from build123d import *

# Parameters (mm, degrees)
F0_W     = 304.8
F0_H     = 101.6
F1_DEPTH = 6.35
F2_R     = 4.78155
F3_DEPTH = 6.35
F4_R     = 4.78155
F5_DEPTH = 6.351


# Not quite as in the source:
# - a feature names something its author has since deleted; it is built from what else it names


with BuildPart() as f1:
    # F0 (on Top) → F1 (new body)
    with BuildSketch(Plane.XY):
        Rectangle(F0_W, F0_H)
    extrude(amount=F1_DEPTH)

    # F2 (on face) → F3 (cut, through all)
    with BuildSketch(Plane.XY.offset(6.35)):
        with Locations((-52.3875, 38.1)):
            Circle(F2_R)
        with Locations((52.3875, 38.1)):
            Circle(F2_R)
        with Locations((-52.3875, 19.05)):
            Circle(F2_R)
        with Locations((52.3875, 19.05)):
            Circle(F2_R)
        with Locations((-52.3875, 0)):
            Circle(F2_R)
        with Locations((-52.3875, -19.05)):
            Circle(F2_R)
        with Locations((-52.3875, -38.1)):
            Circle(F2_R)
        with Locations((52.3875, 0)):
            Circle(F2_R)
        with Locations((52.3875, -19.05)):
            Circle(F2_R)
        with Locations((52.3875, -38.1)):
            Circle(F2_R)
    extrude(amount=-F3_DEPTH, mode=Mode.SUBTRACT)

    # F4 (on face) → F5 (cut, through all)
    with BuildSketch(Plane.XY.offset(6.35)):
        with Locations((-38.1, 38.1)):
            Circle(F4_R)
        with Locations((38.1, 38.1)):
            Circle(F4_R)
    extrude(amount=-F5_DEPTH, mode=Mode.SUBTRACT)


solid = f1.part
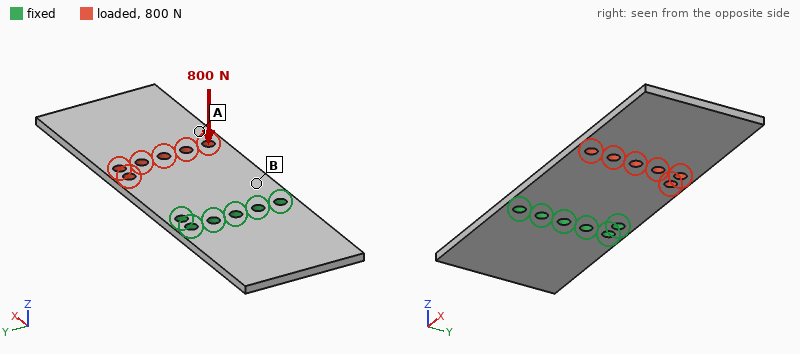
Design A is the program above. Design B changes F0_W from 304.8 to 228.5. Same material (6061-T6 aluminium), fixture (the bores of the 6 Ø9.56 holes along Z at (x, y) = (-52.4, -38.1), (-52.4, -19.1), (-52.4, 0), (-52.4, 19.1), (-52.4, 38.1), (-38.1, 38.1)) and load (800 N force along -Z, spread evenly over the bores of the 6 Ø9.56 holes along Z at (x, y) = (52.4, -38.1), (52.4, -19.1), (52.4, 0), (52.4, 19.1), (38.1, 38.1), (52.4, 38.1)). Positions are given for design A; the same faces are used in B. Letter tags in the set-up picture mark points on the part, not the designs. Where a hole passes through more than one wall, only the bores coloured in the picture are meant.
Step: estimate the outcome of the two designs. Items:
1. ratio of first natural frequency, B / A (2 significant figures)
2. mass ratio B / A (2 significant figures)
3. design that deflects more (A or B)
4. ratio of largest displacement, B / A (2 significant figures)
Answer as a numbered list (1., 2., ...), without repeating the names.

1. 1.6
2. 0.74
3. A
4. 0.77
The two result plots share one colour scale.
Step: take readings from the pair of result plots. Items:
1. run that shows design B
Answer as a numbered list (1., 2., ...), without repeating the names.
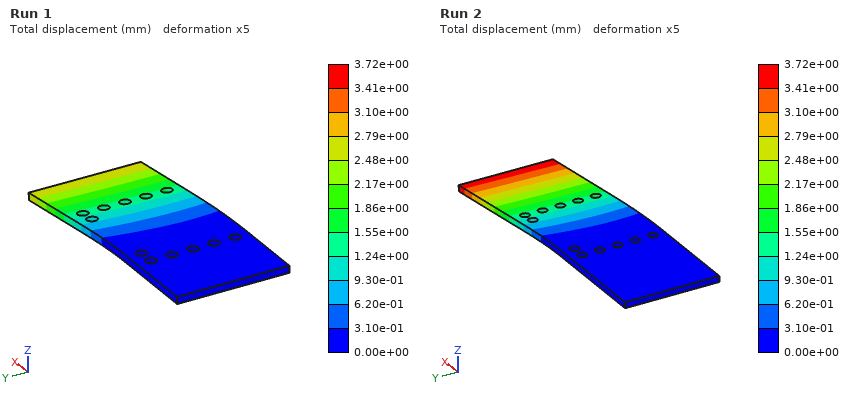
1. Run 1
